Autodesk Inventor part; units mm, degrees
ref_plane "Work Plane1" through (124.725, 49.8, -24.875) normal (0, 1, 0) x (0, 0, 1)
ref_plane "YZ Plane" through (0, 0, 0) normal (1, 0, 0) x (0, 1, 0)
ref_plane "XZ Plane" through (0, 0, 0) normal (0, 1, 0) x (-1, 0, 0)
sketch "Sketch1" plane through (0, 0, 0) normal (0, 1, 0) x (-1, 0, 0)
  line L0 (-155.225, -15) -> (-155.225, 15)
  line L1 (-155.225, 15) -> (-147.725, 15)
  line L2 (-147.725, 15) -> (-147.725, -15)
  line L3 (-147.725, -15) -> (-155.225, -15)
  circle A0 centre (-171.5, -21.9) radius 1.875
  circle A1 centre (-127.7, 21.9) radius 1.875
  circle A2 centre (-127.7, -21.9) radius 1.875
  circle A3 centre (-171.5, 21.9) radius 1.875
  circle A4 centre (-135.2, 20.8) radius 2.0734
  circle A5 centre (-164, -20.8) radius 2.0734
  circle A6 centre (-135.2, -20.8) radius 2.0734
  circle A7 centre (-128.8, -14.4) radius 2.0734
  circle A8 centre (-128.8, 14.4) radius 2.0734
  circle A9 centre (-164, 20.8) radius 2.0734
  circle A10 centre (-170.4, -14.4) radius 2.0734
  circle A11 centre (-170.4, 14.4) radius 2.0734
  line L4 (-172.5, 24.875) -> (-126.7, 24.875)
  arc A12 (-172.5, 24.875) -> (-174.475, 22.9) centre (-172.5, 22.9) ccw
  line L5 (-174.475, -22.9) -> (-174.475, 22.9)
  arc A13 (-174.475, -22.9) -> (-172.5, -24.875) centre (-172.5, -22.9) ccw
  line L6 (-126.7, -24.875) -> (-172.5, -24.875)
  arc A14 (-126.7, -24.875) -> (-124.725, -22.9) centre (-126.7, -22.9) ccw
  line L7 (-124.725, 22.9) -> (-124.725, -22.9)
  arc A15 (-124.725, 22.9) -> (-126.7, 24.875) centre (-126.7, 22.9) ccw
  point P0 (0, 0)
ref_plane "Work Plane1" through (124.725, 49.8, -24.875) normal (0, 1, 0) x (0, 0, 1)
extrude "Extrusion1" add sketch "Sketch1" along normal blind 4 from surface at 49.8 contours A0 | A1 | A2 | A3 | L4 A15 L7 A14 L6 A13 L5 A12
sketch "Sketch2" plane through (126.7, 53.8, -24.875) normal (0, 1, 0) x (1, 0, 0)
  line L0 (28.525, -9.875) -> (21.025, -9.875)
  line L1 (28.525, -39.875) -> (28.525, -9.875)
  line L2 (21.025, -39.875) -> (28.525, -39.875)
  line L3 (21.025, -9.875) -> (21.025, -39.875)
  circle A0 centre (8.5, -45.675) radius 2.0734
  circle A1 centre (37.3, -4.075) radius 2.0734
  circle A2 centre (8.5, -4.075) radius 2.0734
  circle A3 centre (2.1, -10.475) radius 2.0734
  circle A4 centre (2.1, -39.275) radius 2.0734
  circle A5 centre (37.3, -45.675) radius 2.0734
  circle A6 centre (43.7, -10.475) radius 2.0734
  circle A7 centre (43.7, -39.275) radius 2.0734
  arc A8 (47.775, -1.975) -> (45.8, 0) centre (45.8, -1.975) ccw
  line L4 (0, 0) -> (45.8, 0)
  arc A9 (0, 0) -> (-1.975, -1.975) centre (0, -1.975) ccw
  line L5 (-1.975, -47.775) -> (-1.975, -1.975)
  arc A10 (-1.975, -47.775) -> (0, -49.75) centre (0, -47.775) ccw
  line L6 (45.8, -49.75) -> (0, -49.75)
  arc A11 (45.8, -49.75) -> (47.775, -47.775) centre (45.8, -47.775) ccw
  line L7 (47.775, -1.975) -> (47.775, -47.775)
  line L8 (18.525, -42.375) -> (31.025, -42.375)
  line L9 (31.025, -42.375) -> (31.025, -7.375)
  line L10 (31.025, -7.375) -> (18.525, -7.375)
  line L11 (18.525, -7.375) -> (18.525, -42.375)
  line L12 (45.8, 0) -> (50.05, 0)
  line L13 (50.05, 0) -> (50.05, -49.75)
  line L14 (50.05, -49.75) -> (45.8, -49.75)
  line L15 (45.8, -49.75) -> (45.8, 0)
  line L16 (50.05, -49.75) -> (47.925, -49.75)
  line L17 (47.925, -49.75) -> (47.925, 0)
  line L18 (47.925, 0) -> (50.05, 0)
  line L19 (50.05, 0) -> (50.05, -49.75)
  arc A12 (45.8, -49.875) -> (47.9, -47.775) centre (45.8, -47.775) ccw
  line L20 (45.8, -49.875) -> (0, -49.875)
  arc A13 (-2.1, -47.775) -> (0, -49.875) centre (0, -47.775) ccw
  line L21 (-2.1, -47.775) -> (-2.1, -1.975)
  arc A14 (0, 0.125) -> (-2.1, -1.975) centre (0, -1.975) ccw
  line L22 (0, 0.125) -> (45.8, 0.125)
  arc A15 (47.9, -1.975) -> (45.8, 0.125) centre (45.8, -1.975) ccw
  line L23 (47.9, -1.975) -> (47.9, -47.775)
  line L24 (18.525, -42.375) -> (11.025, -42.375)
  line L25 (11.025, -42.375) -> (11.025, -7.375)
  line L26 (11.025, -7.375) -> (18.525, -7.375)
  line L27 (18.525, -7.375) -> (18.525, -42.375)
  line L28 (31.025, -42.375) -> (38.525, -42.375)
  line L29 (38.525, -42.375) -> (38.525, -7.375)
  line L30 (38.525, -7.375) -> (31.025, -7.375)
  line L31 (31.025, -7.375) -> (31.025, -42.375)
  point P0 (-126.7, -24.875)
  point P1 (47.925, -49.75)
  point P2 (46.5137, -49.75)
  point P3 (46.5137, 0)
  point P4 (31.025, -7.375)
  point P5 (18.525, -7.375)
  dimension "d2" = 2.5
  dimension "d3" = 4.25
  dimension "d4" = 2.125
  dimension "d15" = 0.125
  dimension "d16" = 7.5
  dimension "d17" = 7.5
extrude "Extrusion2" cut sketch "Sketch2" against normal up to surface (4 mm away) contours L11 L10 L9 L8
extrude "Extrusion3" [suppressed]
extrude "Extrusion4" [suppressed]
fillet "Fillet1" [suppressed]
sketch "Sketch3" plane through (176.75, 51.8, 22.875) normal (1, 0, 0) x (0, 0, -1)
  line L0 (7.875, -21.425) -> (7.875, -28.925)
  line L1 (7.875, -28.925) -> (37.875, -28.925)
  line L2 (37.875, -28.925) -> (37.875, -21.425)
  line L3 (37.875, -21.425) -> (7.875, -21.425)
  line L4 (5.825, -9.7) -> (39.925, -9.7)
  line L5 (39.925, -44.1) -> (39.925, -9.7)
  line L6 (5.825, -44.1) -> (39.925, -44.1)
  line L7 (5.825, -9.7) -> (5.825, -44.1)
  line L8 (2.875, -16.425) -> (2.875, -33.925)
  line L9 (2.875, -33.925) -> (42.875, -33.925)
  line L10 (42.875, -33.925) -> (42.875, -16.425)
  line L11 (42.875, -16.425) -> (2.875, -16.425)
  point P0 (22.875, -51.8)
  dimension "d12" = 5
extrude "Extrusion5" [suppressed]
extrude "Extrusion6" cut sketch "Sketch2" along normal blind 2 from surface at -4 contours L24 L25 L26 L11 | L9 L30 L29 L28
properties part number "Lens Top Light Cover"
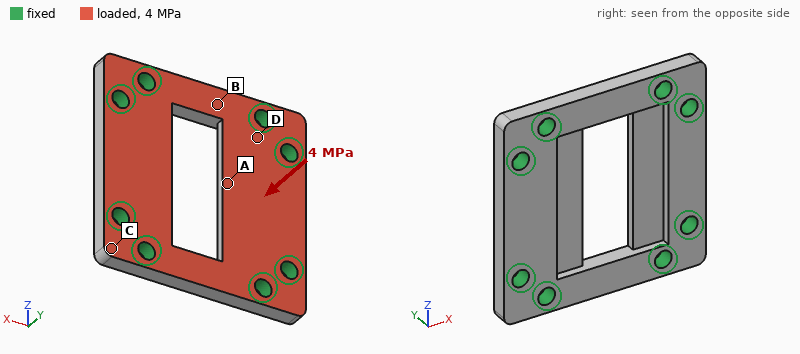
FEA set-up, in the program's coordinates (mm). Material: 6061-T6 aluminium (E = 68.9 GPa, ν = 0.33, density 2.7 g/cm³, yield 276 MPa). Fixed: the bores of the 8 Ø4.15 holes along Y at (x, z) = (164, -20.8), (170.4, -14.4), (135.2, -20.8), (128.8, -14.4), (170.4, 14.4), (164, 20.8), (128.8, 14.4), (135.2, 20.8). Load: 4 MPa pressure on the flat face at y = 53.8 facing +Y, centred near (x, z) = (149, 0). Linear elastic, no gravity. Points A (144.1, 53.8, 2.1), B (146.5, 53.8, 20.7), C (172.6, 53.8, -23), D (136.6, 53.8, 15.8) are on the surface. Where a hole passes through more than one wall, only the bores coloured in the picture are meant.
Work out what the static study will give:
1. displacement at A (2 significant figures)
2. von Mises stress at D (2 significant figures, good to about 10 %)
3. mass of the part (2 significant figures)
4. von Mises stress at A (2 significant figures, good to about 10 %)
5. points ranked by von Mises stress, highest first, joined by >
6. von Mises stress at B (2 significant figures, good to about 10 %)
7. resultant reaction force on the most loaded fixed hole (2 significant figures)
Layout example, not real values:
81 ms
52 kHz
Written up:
0.14 mm
100 MPa
18 g
77 MPa
D > A > B > C
45 MPa
1.1 kN
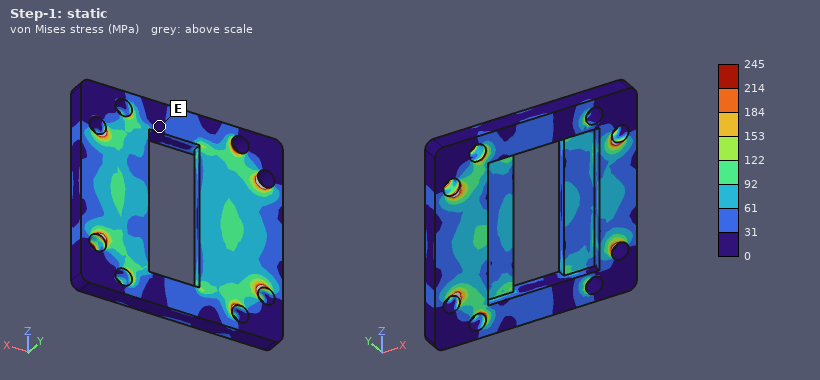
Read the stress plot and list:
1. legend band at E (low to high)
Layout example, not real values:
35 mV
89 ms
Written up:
0 to 31 MPa
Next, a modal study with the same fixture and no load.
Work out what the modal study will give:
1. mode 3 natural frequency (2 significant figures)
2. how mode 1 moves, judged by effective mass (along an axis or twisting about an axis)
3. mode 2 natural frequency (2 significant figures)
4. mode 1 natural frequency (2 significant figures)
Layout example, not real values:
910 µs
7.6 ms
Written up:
26 kHz
along Y
17 kHz
15 kHz
